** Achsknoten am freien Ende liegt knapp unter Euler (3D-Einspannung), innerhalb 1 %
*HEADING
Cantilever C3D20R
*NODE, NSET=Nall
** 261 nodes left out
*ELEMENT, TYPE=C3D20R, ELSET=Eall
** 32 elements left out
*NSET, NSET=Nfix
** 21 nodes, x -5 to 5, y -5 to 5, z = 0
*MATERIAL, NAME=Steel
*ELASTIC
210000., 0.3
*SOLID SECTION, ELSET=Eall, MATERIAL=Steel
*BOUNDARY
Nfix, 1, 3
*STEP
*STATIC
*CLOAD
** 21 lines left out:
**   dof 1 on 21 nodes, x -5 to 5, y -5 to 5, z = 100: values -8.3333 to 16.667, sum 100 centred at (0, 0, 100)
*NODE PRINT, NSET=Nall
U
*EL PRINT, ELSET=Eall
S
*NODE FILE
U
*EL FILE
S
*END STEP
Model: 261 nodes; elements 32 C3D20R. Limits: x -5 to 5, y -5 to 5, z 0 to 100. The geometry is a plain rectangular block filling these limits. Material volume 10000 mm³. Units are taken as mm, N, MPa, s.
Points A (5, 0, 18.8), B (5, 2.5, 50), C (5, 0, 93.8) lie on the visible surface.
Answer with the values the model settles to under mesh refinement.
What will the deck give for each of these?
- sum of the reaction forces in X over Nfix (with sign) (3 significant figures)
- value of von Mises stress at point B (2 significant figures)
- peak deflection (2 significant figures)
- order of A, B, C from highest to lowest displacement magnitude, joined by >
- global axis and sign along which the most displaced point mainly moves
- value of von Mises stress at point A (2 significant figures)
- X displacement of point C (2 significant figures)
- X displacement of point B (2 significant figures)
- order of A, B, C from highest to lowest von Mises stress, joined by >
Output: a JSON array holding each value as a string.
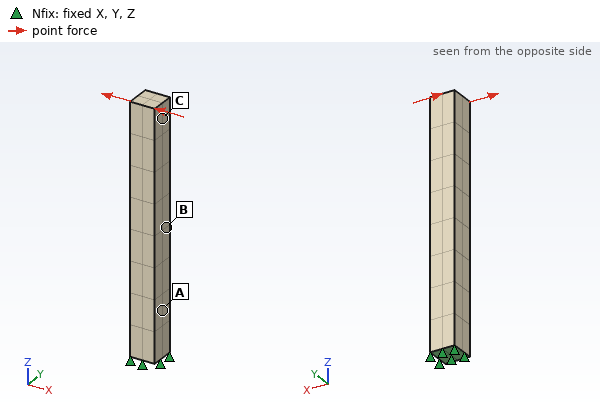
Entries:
["-100 N", "30 MPa", "0.19 mm", "C > B > A", "+X", "49 MPa", "0.17 mm", "0.060 mm", "A > B > C"]
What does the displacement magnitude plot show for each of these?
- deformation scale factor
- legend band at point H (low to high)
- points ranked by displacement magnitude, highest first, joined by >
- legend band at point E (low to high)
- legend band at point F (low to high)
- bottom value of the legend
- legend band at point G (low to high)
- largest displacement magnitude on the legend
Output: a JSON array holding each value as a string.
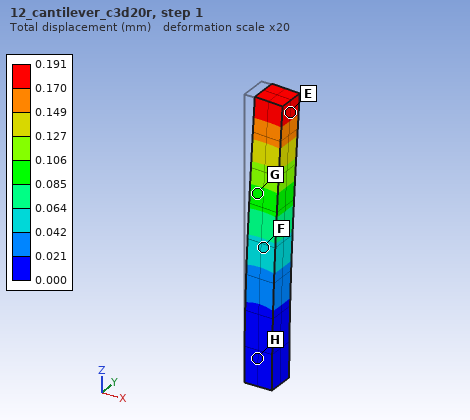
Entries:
["20", "0.000 to 0.021 mm", "E > G > F > H", "0.170 to 0.191 mm", "0.042 to 0.064 mm", "0.000 mm", "0.085 to 0.106 mm", "0.191 mm"]
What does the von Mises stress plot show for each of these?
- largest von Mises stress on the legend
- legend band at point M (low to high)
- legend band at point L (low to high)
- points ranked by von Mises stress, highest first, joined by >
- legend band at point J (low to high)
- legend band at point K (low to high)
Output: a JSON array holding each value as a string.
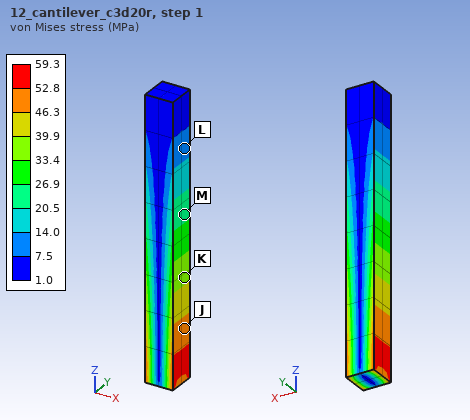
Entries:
["59.3 MPa", "20.5 to 26.9 MPa", "7.5 to 14.0 MPa", "J > K > M > L", "46.3 to 52.8 MPa", "33.4 to 39.9 MPa"]
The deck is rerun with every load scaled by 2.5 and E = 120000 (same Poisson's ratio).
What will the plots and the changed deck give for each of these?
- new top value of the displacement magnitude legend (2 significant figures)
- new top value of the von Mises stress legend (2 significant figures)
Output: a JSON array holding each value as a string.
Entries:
["0.84 mm", "150 MPa"]
